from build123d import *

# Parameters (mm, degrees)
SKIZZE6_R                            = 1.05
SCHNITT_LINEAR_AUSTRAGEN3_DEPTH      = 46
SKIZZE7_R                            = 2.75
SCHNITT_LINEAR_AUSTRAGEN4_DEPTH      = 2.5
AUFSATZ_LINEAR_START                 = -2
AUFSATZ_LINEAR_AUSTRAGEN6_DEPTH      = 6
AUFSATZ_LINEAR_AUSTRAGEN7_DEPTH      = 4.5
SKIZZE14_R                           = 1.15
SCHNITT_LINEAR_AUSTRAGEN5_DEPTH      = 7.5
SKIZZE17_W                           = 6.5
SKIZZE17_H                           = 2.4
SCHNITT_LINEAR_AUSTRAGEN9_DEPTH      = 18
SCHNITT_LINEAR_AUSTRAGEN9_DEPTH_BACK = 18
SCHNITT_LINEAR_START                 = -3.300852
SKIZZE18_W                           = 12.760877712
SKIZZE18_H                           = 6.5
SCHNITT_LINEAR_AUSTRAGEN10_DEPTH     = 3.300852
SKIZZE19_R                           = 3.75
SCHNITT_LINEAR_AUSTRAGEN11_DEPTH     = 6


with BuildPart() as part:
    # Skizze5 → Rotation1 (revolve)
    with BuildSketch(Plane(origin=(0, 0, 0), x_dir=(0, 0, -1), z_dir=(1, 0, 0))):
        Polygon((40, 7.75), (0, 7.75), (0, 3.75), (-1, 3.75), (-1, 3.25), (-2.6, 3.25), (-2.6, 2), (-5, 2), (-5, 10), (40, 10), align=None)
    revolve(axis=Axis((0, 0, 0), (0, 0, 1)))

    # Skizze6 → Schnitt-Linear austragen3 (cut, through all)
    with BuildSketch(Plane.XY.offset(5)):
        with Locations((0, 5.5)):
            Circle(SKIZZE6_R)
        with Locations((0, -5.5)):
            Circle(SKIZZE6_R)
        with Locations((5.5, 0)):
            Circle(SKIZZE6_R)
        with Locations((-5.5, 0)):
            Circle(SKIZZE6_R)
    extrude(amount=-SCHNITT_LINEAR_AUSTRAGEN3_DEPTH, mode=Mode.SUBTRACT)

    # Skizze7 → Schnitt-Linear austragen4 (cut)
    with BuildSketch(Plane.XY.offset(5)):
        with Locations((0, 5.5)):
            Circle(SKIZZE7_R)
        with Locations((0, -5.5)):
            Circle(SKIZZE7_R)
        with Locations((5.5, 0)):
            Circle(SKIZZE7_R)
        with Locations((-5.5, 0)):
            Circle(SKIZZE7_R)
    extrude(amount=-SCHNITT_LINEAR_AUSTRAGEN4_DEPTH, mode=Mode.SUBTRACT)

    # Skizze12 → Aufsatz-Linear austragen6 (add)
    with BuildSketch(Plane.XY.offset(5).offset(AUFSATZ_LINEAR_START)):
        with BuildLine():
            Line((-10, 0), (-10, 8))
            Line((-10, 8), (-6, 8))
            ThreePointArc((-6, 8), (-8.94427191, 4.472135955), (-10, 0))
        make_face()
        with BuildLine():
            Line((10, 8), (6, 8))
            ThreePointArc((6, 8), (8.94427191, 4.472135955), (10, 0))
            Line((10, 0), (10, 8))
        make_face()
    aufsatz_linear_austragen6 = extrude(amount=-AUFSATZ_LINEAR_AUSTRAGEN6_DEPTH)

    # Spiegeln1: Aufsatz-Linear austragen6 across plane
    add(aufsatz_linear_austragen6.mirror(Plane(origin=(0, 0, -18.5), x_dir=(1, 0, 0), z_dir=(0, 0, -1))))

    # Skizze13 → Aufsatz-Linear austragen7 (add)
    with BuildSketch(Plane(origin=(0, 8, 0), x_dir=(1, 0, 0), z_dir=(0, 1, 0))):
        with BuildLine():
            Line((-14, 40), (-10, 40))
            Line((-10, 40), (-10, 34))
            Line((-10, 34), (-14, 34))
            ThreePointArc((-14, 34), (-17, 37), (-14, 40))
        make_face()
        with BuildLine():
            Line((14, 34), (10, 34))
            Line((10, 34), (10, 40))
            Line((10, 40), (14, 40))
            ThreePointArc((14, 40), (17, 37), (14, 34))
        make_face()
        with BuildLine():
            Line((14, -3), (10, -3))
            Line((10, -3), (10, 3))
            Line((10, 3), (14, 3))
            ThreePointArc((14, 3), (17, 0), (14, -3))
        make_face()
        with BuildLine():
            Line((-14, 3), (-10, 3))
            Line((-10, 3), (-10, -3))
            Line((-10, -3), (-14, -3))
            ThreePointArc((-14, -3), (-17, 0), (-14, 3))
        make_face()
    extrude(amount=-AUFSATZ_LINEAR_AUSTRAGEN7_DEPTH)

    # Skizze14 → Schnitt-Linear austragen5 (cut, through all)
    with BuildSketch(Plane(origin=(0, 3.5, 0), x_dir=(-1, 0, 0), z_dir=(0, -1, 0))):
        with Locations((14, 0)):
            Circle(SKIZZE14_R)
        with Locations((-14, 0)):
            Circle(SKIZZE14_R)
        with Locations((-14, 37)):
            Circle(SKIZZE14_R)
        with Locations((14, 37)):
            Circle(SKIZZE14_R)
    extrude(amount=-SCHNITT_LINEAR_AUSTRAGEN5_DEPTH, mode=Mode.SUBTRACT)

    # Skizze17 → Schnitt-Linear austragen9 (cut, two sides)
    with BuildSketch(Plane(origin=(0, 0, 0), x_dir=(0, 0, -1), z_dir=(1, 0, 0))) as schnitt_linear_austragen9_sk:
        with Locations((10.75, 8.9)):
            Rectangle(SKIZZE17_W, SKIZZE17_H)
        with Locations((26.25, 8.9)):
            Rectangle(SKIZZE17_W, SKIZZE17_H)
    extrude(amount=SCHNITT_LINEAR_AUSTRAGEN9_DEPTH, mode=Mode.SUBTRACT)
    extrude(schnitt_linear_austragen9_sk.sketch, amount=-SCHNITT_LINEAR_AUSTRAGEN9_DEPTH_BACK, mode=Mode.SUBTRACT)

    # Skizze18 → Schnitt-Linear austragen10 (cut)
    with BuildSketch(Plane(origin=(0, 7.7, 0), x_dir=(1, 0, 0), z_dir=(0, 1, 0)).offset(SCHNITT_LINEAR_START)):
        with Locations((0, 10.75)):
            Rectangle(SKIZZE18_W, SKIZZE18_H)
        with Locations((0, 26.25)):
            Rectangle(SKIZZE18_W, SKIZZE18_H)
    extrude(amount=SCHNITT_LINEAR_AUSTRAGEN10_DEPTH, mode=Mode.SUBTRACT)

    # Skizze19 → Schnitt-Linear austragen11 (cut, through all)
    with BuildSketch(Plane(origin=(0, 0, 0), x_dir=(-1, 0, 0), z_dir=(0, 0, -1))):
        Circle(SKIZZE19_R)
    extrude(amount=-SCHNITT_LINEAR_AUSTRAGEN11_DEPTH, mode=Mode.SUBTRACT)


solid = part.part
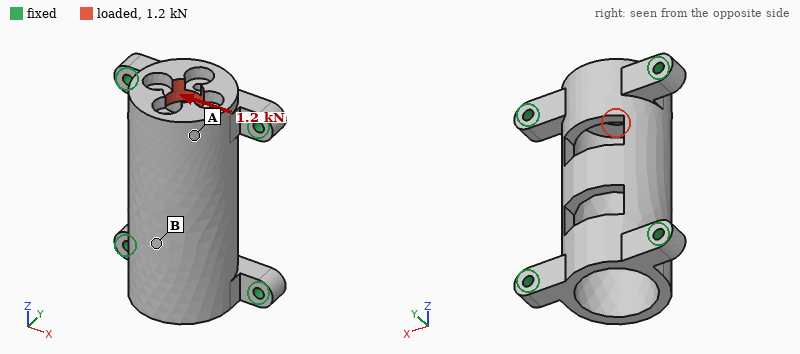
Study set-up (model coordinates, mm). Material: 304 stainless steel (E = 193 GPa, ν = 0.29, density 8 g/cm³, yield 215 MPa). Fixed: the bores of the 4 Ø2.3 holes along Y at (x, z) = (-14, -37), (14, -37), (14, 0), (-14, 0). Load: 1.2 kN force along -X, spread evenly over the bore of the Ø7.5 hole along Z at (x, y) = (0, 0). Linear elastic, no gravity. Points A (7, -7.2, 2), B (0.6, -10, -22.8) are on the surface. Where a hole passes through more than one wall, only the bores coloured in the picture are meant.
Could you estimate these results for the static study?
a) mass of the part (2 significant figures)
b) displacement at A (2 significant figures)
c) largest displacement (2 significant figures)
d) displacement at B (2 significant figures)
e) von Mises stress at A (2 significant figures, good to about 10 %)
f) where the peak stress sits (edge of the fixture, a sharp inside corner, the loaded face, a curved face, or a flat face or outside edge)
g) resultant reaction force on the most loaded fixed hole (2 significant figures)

52 g
4.8 µm
5.5 µm
2.1 µm
15 MPa
a curved face
630 N
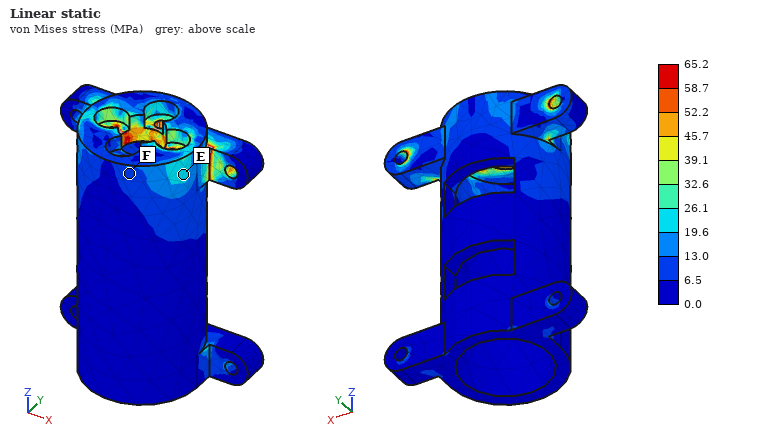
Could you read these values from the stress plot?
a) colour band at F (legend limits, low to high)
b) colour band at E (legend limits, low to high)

6.5 to 13.0 MPa
19.6 to 26.1 MPa
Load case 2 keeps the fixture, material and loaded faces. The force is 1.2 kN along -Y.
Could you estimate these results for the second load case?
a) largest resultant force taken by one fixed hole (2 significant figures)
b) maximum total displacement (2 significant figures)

630 N
6.8 µm
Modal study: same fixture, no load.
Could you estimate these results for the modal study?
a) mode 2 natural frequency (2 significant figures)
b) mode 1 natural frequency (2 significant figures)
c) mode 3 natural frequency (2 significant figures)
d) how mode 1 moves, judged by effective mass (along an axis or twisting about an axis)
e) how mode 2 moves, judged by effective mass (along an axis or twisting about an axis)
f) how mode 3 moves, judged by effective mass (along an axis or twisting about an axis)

14 kHz
11 kHz
16 kHz
along X
along Z
along Y
